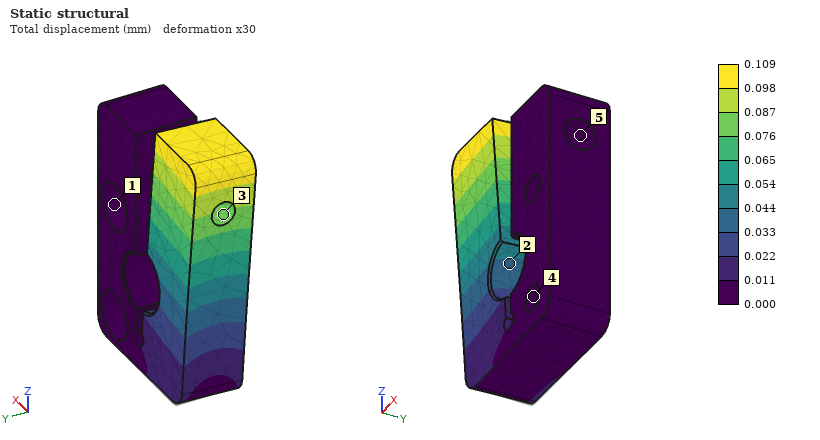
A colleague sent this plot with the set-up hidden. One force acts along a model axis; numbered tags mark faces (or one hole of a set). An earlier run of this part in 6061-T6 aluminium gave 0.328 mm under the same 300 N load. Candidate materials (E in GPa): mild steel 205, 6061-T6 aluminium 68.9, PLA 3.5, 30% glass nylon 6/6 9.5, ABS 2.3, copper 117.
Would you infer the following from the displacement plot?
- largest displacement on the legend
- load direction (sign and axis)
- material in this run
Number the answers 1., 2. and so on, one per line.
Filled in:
1. 0.109 mm
2. -Y
3. mild steel
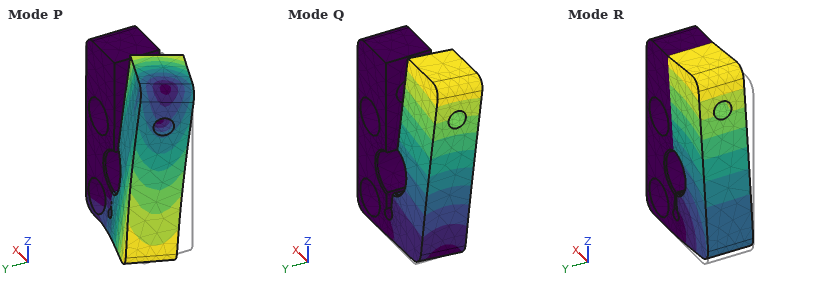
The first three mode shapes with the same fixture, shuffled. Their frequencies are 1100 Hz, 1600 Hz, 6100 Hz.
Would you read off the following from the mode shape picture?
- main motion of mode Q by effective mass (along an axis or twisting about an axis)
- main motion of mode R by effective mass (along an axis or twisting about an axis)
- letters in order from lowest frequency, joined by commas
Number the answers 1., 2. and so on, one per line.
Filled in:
1. along Y
2. along X
3. R, Q, P
